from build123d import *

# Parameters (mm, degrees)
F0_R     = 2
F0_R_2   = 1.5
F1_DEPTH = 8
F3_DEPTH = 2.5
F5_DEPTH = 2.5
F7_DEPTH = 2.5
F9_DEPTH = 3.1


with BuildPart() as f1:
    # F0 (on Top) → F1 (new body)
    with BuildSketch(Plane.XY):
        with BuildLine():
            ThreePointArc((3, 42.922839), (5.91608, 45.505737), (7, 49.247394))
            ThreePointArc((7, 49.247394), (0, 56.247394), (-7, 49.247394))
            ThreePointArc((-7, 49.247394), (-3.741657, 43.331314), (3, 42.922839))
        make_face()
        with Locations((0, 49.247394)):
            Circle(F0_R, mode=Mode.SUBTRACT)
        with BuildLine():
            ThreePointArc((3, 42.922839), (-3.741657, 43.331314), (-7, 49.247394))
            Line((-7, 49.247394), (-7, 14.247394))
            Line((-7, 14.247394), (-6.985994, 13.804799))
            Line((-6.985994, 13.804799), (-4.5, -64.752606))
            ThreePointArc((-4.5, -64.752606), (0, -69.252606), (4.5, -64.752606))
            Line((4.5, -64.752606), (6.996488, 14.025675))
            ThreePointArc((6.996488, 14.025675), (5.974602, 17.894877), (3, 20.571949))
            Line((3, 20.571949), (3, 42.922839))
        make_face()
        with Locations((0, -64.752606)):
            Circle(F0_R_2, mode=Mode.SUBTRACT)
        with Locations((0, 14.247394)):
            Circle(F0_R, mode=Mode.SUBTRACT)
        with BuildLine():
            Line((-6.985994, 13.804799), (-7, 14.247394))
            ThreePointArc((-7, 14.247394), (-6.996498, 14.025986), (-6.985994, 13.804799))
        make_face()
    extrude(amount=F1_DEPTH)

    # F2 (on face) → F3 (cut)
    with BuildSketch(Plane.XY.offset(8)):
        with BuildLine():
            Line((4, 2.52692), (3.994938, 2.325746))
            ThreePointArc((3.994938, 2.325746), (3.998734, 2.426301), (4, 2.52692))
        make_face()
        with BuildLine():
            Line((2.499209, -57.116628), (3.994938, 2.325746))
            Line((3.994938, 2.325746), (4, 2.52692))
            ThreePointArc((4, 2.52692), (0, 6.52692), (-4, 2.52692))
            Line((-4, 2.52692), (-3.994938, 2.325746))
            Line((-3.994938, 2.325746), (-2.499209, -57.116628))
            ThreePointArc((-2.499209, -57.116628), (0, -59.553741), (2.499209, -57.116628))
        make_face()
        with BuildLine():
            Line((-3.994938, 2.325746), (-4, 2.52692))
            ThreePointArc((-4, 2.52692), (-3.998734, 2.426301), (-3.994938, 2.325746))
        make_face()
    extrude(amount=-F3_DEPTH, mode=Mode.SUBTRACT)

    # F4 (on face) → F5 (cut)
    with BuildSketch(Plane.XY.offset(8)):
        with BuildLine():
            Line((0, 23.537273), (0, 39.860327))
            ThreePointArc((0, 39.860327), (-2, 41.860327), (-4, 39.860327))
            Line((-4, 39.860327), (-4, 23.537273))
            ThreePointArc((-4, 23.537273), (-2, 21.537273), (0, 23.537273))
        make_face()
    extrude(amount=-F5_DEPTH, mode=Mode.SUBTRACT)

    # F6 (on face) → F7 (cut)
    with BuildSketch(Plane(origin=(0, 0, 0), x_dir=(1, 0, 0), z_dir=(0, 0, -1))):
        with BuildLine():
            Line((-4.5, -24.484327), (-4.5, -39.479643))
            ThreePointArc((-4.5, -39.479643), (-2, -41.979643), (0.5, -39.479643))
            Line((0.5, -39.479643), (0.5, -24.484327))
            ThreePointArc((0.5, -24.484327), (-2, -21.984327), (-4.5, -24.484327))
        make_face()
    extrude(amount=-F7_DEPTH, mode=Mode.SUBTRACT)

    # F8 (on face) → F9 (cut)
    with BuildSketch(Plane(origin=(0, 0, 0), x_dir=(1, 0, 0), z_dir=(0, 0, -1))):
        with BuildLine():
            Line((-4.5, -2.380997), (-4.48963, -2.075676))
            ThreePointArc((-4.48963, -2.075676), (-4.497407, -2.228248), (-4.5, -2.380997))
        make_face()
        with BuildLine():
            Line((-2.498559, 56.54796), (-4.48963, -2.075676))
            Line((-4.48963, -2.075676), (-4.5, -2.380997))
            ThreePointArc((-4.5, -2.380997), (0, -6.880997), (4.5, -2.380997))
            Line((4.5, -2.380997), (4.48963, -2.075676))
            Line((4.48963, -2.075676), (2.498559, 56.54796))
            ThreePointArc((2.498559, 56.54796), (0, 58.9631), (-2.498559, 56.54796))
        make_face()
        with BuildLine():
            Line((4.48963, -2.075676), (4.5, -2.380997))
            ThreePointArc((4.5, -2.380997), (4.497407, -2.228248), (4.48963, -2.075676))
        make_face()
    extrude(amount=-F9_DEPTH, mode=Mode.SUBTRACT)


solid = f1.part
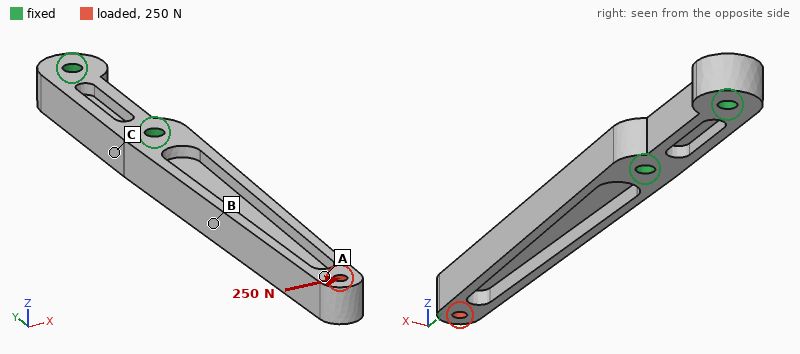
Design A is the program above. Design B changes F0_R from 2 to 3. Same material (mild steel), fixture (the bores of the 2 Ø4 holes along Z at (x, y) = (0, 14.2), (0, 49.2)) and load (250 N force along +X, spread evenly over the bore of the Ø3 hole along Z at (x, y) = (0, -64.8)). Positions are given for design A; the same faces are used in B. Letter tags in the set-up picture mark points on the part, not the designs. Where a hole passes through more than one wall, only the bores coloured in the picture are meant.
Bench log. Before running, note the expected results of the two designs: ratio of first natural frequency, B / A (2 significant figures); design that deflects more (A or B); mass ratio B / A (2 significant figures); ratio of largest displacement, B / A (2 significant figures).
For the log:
1.0
A
0.97
0.91
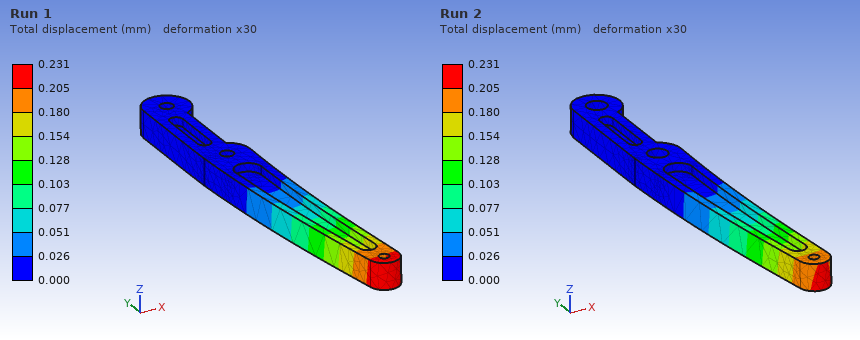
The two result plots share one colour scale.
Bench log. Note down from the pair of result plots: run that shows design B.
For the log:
Run 2
